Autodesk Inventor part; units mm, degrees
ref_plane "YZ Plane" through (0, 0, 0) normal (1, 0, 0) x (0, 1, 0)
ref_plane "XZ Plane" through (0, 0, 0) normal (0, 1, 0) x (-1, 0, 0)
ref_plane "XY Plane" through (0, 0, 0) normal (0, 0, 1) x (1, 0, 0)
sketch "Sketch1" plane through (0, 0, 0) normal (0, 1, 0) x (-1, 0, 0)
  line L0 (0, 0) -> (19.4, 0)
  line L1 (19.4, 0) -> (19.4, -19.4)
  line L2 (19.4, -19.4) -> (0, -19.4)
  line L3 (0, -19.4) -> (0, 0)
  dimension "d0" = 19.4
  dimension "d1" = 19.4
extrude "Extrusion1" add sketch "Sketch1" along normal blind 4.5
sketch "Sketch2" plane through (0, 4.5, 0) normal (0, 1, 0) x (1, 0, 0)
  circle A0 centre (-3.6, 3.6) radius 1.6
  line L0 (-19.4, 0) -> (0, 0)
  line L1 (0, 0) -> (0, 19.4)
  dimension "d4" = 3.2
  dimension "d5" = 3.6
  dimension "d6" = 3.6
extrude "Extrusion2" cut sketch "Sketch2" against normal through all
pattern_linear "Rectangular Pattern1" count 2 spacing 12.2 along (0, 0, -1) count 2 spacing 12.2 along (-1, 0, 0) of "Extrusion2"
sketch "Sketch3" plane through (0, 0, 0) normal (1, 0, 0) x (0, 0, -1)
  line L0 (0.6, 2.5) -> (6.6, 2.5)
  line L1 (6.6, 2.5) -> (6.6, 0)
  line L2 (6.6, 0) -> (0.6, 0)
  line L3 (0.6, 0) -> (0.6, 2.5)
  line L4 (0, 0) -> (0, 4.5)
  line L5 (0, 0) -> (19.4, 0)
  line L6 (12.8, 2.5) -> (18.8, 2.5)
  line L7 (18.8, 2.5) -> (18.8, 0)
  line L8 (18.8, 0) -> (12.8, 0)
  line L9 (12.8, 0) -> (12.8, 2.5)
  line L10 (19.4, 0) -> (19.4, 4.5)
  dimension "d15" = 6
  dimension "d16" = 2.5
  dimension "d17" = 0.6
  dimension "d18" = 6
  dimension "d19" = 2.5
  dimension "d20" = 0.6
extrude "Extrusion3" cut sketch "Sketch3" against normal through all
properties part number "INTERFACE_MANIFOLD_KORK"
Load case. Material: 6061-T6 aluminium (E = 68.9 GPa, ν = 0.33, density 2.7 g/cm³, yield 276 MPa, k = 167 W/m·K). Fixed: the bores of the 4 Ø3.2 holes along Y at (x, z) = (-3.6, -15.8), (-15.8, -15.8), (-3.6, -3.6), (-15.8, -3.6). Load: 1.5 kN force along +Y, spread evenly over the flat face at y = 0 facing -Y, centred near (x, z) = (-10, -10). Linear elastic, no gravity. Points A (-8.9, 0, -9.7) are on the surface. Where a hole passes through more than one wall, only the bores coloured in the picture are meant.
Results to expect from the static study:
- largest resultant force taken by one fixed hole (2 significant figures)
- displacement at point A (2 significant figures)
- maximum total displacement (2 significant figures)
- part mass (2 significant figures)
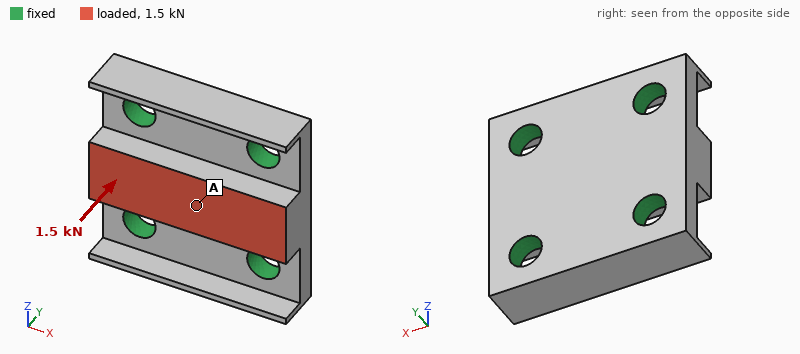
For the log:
400 N
7.0 µm
7.0 µm
2.8 g
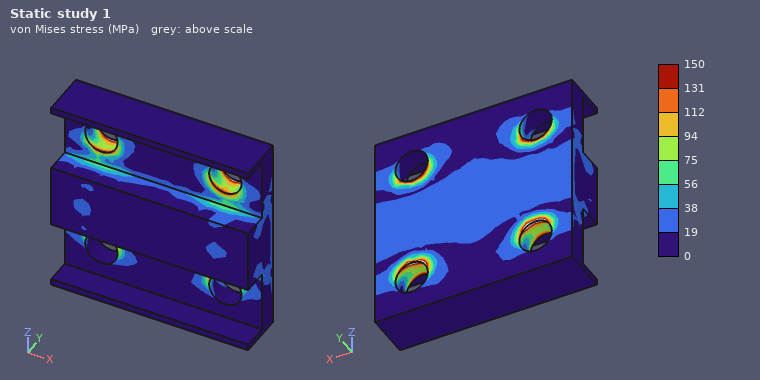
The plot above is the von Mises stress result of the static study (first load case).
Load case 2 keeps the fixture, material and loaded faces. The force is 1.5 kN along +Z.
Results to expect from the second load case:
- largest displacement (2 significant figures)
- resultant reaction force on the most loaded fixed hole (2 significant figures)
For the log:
7.9 µm
480 N
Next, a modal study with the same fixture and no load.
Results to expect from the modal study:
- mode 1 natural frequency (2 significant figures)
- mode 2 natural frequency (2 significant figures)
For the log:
58 kHz
58 kHz
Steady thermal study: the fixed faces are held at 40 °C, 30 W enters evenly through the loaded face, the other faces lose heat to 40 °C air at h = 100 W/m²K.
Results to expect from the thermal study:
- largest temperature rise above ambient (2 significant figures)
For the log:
13 K
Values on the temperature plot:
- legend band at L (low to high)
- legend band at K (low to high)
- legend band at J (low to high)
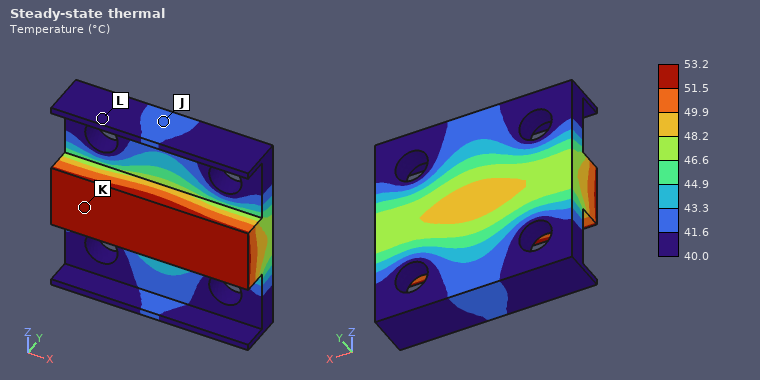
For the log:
40.0 to 41.6 °C
51.5 to 53.2 °C
41.6 to 43.3 °C
